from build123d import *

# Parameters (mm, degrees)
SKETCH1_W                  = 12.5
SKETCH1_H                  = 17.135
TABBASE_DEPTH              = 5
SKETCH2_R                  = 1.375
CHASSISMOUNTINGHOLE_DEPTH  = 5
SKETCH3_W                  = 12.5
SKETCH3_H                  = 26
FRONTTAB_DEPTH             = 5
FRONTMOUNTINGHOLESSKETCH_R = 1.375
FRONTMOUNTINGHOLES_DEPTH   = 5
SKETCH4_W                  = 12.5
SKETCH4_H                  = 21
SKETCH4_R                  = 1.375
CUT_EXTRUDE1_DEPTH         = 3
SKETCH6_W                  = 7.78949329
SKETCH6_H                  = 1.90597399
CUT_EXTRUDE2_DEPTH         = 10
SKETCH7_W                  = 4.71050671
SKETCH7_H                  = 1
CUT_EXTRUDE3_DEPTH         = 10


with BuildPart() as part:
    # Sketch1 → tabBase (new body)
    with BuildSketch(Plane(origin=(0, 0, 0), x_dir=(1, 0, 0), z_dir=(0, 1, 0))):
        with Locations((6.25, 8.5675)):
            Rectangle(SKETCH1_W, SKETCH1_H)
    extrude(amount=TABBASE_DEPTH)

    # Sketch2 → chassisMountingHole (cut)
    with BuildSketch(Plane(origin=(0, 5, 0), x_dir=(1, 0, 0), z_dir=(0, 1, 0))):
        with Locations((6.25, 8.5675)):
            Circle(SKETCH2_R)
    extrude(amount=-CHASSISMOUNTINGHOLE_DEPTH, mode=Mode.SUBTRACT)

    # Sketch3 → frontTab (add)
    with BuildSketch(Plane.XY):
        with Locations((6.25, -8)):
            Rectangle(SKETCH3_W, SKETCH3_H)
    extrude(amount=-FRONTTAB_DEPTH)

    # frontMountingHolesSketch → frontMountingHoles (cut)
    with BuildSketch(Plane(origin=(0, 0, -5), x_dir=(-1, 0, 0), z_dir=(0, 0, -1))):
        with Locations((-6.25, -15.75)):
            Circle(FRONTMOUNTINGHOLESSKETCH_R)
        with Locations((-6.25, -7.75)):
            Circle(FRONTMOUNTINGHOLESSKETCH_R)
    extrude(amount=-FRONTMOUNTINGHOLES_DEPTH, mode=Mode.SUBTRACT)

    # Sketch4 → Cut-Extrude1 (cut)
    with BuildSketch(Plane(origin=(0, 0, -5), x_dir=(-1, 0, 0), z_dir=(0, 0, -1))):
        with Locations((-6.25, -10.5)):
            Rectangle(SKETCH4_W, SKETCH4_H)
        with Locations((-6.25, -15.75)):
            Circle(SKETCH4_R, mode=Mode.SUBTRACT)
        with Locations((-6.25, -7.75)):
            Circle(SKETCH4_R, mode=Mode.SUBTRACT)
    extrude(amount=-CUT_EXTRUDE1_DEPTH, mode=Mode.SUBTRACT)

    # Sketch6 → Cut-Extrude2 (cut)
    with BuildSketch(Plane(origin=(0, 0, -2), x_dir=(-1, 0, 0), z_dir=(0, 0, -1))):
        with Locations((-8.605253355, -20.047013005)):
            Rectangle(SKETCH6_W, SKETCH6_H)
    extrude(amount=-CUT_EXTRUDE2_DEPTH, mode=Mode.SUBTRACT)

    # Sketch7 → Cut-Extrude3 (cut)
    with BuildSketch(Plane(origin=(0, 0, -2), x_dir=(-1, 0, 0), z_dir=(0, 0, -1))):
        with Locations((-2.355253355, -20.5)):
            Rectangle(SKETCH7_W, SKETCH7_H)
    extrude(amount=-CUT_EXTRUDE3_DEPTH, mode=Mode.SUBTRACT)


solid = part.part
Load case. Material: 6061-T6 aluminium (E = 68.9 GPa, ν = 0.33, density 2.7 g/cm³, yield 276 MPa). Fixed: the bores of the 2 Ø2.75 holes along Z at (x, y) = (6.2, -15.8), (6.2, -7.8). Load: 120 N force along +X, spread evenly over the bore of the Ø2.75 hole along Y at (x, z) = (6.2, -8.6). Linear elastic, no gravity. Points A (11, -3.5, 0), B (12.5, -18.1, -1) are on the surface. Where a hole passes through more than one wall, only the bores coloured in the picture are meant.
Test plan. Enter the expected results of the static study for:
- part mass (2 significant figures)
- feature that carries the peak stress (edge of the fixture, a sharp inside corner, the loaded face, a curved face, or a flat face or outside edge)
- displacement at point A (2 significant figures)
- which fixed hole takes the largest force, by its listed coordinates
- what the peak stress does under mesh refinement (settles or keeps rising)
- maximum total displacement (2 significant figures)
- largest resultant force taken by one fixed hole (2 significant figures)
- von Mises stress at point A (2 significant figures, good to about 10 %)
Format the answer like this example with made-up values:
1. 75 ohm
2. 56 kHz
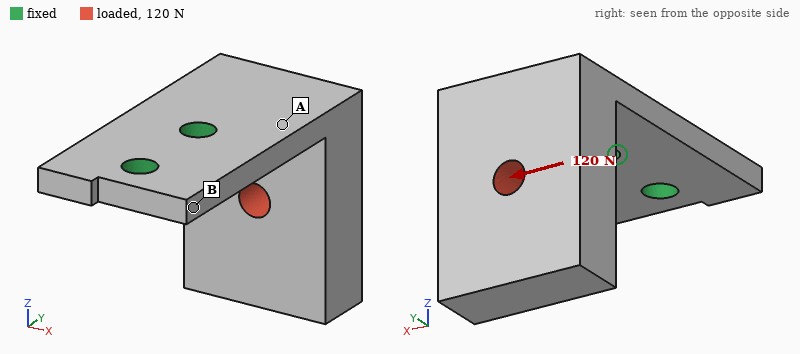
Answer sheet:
1. 4.1 g
2. edge of the fixture
3. 0.020 mm
4. (6.2, -7.8)
5. keeps rising
6. 0.12 mm
7. 210 N
8. 46 MPa
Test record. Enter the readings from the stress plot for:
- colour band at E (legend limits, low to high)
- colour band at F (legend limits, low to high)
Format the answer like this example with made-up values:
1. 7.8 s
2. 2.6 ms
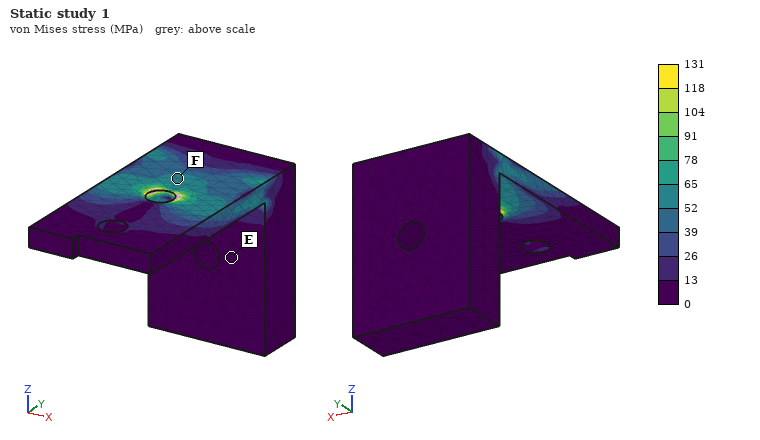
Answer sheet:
1. 0 to 13 MPa
2. 52 to 65 MPa
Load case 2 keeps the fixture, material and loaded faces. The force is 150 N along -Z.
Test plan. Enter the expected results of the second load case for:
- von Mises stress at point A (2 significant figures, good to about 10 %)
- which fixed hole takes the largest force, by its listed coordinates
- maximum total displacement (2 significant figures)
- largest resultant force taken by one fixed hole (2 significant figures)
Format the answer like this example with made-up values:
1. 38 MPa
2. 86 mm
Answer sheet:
1. 95 MPa
2. (6.2, -7.8)
3. 0.23 mm
4. 190 N
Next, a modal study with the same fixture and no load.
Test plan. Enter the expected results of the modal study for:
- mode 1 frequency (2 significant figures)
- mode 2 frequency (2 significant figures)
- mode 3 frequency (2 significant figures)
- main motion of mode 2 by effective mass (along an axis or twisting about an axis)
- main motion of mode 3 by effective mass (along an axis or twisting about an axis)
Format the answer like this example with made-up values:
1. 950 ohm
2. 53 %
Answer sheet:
1. 2300 Hz
2. 3500 Hz
3. 10 kHz
4. along X
5. along Z
